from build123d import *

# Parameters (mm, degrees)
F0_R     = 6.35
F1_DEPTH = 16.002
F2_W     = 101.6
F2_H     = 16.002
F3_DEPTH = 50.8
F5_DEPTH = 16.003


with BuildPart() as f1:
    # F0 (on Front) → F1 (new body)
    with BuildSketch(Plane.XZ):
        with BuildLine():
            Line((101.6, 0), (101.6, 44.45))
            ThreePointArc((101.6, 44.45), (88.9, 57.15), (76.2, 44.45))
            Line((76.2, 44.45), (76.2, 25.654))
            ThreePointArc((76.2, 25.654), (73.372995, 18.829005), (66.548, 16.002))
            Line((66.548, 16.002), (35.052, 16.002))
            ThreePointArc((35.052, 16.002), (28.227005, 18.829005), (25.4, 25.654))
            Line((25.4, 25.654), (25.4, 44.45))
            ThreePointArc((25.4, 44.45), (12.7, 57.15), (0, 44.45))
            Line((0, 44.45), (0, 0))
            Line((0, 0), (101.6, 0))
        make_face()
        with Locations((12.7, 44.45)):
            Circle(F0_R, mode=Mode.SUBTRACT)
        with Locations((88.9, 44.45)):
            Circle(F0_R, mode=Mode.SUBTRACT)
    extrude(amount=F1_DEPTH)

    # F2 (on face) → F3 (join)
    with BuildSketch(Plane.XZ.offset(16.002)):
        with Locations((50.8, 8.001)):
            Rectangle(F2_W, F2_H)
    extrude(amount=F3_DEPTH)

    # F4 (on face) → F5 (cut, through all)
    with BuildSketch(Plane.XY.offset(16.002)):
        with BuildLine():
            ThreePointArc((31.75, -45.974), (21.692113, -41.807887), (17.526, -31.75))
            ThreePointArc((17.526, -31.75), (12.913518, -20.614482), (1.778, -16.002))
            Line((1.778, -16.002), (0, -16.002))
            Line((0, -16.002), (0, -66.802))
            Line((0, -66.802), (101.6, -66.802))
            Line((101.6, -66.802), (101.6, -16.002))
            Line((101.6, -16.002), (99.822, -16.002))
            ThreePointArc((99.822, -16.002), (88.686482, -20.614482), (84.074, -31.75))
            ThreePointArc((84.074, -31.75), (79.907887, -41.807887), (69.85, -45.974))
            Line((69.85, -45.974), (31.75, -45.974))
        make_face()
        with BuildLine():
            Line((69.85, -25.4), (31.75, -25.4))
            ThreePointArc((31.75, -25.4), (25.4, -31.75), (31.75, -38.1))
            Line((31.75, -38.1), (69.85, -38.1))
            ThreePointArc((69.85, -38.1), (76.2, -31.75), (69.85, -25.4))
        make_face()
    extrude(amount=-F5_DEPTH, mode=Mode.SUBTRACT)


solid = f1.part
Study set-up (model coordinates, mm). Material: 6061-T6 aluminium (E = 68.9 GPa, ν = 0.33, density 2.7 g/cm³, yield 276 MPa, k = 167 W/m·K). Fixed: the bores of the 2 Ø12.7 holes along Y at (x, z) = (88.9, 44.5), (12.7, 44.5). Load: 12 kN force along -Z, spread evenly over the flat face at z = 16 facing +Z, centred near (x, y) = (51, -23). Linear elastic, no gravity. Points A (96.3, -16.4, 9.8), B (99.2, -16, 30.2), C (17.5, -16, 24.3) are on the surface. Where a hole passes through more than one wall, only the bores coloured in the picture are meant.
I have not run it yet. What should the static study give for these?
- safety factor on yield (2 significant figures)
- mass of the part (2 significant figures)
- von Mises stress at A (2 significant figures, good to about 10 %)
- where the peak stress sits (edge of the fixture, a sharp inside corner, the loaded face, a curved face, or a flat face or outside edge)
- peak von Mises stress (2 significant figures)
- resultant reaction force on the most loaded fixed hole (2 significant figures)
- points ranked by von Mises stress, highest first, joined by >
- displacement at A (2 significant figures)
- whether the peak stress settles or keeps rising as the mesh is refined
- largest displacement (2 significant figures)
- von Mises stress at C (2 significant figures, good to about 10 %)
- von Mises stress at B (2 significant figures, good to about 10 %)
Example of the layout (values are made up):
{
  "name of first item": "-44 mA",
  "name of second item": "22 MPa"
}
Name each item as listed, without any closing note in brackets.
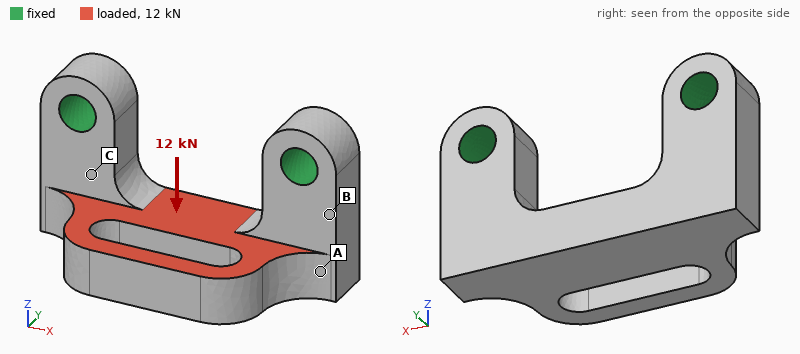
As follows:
{
  "safety factor on yield": "1.5",
  "mass of the part": "210 g",
  "von Mises stress at A": "25 MPa",
  "where the peak stress sits": "a curved face",
  "peak von Mises stress": "180 MPa",
  "resultant reaction force on the most loaded fixed hole": "6.5 kN",
  "points ranked by von Mises stress, highest first, joined by >": "C > B > A",
  "displacement at A": "0.080 mm",
  "whether the peak stress settles or keeps rising as the mesh is refined": "settles",
  "largest displacement": "0.33 mm",
  "von Mises stress at C": "110 MPa",
  "von Mises stress at B": "72 MPa"
}
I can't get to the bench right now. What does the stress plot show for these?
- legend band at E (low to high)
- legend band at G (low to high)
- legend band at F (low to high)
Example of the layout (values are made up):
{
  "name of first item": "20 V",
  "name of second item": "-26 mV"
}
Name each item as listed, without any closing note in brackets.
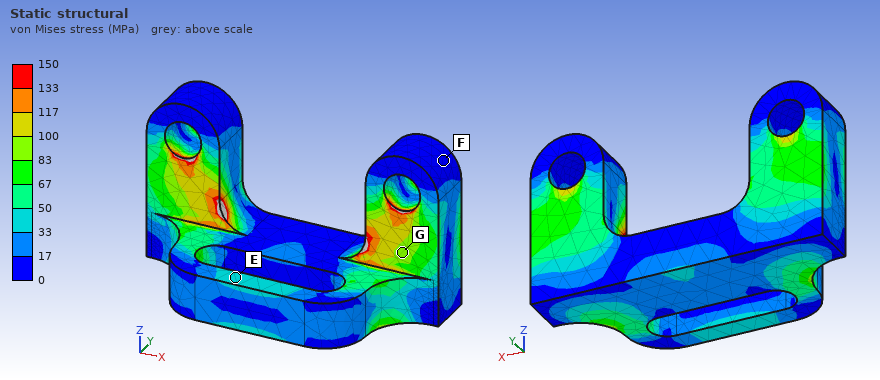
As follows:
{
  "legend band at E": "33 to 50 MPa",
  "legend band at G": "83 to 100 MPa",
  "legend band at F": "0 to 17 MPa"
}
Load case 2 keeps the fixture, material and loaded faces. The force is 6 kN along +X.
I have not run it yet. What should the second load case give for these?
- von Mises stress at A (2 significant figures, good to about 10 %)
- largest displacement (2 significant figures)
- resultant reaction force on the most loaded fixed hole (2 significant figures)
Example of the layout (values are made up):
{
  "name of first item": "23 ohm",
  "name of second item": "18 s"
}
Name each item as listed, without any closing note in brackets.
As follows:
{
  "von Mises stress at A": "7.2 MPa",
  "largest displacement": "68 µm",
  "resultant reaction force on the most loaded fixed hole": "3.2 kN"
}
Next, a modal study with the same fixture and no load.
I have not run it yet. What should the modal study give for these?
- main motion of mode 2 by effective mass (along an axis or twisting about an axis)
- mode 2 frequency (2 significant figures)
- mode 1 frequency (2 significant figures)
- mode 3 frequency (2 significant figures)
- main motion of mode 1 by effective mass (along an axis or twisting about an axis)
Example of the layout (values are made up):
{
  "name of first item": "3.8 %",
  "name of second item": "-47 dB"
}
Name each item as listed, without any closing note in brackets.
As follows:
{
  "main motion of mode 2 by effective mass": "along X",
  "mode 2 frequency": "5600 Hz",
  "mode 1 frequency": "3100 Hz",
  "mode 3 frequency": "6900 Hz",
  "main motion of mode 1 by effective mass": "along Y"
}
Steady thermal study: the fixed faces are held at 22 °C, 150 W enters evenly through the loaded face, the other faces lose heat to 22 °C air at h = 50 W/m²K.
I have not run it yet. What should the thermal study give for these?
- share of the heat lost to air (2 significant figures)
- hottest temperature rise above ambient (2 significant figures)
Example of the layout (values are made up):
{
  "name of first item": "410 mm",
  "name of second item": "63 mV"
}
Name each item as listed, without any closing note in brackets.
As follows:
{
  "share of the heat lost to air": "14 %",
  "hottest temperature rise above ambient": "61 K"
}
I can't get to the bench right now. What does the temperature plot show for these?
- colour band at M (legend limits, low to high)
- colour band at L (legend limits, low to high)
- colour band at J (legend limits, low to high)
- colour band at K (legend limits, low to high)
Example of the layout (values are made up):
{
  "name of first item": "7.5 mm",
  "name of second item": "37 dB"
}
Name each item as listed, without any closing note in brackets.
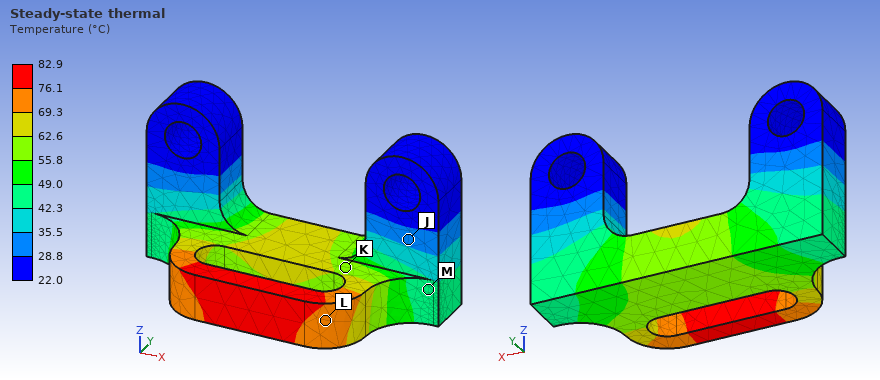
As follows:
{
  "colour band at M": "42.3 to 49.0 °C",
  "colour band at L": "69.3 to 76.1 °C",
  "colour band at J": "28.8 to 35.5 °C",
  "colour band at K": "55.8 to 62.6 °C"
}
